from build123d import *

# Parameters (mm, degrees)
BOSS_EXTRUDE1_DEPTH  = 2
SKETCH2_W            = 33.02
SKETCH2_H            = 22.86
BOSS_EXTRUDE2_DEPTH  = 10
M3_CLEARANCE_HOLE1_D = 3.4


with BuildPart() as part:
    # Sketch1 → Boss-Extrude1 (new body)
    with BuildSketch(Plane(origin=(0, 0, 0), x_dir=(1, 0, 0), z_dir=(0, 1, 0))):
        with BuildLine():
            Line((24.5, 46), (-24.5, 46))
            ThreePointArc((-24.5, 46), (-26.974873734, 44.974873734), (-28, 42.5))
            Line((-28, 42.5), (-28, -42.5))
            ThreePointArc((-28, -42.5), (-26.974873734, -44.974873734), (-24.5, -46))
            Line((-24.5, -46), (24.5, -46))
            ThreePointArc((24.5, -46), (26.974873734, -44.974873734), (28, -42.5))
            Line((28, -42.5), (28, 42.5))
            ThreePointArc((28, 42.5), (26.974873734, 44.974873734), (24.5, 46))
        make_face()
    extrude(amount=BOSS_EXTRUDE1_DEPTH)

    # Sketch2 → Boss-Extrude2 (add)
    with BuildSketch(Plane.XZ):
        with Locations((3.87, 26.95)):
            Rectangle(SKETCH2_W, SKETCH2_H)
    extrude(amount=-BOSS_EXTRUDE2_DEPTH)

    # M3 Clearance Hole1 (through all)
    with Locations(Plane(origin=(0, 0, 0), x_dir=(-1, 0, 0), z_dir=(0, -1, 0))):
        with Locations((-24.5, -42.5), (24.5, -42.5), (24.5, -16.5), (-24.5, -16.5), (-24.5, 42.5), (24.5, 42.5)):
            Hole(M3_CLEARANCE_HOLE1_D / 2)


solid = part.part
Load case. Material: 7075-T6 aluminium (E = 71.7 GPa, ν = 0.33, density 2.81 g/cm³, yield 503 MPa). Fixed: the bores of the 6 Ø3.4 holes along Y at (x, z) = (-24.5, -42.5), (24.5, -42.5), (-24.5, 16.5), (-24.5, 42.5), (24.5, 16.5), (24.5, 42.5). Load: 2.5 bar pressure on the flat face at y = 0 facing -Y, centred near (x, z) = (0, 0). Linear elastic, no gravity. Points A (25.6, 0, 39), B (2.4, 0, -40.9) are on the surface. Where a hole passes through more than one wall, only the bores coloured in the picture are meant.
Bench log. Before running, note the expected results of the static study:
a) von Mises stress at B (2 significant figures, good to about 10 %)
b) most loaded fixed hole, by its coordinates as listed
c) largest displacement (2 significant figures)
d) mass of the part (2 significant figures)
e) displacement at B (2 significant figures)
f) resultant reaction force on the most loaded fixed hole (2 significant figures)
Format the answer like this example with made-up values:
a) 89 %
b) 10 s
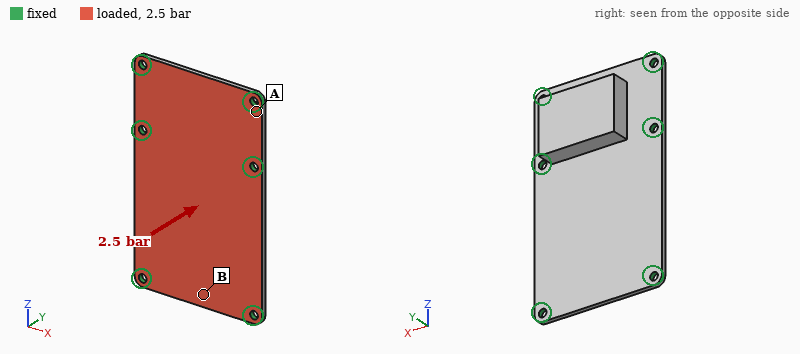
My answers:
a) 46 MPa
b) (24.5, 16.5)
c) 0.24 mm
d) 46 g
e) 0.11 mm
f) 460 N
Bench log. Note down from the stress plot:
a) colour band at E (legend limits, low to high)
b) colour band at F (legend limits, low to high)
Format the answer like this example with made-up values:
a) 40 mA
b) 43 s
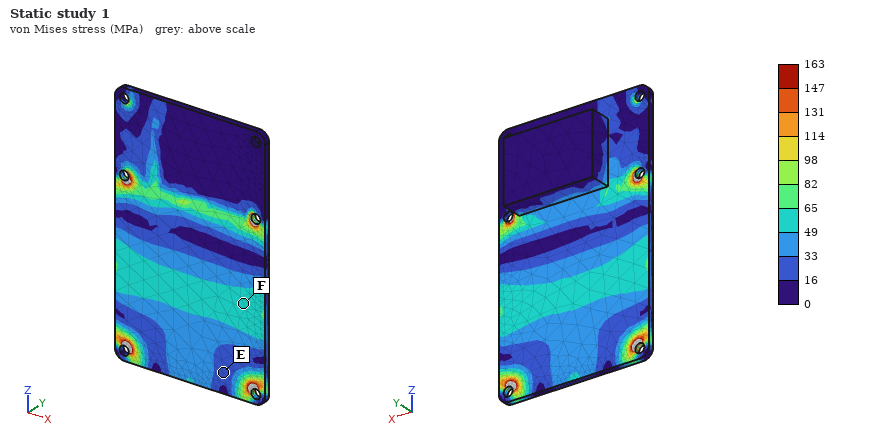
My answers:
a) 16 to 33 MPa
b) 49 to 65 MPa
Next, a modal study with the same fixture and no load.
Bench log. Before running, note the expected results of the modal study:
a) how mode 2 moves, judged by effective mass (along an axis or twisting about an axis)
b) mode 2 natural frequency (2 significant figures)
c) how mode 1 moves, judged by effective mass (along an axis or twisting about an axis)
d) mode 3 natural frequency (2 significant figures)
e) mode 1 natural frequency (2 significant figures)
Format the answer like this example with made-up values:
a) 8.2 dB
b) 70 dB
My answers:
a) twisting about Z
b) 3700 Hz
c) along Y
d) 4700 Hz
e) 2600 Hz
